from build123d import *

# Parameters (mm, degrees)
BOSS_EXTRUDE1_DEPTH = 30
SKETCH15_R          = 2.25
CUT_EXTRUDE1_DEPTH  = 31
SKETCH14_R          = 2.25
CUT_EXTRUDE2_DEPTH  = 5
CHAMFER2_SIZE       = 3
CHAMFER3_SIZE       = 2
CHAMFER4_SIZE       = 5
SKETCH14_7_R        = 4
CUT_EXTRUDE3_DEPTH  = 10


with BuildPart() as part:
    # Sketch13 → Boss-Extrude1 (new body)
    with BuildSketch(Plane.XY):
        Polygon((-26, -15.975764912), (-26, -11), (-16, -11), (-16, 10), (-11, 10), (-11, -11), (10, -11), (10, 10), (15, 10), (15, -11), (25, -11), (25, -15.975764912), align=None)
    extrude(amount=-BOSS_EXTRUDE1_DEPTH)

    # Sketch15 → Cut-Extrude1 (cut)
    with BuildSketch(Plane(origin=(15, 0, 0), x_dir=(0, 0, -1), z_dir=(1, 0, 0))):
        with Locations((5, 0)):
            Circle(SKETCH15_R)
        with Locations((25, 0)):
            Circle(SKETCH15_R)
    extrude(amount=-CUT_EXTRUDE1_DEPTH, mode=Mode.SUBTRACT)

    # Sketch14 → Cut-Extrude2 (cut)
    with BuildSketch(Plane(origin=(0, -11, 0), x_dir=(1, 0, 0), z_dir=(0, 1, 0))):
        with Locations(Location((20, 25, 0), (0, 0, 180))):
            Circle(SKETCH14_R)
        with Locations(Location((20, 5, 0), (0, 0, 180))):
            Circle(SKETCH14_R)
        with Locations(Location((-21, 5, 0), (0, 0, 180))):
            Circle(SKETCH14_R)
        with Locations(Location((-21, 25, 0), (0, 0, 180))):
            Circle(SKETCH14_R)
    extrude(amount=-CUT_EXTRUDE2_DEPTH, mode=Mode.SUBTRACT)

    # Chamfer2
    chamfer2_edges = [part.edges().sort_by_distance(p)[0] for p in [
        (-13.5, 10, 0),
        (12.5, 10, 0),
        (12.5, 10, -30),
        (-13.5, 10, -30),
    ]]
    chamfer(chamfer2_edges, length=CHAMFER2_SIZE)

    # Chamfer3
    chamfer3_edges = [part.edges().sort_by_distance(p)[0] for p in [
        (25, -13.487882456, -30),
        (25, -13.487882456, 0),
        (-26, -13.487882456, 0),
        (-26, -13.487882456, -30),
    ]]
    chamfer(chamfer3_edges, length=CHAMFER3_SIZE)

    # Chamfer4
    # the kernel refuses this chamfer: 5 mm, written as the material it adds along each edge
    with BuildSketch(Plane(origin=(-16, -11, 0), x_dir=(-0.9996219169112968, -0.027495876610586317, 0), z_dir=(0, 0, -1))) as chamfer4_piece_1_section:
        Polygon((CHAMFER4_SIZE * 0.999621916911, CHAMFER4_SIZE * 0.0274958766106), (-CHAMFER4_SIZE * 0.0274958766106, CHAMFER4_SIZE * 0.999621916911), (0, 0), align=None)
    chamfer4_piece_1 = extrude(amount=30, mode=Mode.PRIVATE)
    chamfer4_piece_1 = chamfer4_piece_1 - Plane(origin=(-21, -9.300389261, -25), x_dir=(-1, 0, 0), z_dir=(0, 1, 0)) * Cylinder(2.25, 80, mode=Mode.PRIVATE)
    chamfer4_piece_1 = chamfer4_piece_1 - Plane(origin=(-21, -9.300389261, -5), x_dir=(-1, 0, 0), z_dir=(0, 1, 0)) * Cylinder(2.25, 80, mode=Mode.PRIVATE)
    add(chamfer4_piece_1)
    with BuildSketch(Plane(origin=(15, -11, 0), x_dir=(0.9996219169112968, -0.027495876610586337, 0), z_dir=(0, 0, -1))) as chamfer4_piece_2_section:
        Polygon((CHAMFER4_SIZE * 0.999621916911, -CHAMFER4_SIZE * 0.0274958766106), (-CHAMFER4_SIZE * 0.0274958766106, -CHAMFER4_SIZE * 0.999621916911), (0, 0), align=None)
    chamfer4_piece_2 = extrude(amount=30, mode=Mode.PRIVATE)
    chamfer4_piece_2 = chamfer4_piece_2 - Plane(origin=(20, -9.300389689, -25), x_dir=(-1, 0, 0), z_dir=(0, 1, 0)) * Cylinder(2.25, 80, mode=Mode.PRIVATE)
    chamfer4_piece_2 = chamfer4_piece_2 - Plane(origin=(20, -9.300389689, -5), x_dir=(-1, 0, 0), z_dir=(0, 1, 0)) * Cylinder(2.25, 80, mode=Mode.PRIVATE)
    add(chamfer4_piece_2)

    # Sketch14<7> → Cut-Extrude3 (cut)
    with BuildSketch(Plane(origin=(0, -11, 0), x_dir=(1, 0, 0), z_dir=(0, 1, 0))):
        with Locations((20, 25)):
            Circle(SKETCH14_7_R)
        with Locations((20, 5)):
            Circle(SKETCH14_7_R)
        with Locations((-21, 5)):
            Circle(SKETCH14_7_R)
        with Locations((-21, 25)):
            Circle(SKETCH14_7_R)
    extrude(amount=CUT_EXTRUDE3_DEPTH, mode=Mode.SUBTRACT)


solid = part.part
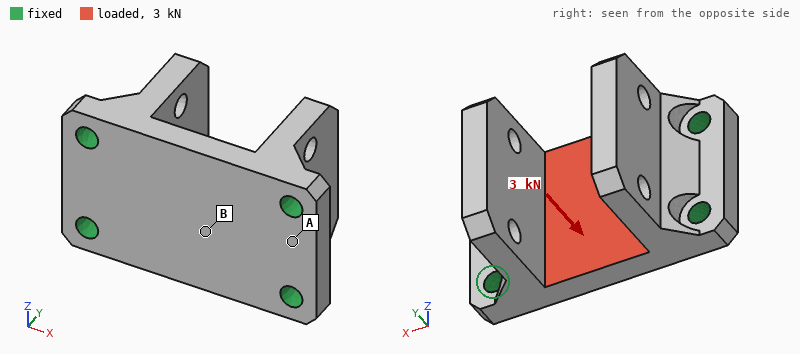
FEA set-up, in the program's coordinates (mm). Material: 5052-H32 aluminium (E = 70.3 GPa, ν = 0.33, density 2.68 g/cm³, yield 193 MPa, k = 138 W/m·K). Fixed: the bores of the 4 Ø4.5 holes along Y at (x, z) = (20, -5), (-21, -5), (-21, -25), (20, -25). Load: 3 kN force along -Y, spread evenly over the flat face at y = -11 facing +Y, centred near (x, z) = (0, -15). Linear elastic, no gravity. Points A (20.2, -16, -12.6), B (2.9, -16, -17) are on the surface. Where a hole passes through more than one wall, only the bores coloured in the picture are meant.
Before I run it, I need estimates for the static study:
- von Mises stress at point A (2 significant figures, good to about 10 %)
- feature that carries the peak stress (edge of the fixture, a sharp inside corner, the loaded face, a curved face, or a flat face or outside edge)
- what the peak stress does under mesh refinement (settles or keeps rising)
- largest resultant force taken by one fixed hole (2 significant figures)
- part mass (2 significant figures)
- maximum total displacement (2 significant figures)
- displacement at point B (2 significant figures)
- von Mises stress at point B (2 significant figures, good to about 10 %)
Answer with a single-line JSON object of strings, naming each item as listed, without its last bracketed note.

{"von Mises stress at point A": "24 MPa", "feature that carries the peak stress": "edge of the fixture", "what the peak stress does under mesh refinement": "keeps rising", "largest resultant force taken by one fixed hole": "750 N", "part mass": "37 g", "maximum total displacement": "55 µm", "displacement at point B": "34 µm", "von Mises stress at point B": "48 MPa"}
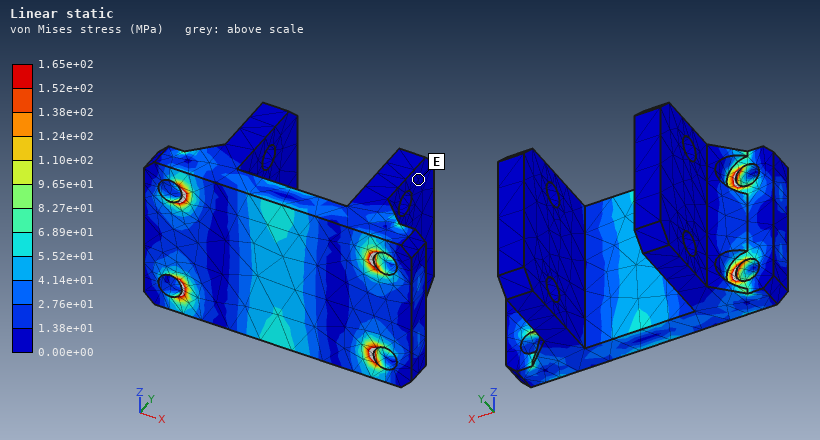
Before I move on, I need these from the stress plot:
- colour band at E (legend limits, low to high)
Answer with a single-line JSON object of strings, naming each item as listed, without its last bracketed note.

{"colour band at E": "0.00e+00 to 1.38e+01 MPa"}
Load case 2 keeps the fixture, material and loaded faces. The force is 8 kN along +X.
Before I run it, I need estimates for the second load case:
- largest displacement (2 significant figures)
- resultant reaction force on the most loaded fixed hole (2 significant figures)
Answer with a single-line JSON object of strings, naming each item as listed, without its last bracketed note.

{"largest displacement": "8.2 µm", "resultant reaction force on the most loaded fixed hole": "2.1 kN"}
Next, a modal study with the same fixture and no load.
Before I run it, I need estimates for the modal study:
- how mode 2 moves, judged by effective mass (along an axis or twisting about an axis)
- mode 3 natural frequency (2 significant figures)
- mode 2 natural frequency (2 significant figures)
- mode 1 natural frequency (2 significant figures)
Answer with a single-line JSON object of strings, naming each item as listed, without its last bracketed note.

{"how mode 2 moves, judged by effective mass": "along X", "mode 3 natural frequency": "14 kHz", "mode 2 natural frequency": "9000 Hz", "mode 1 natural frequency": "7300 Hz"}
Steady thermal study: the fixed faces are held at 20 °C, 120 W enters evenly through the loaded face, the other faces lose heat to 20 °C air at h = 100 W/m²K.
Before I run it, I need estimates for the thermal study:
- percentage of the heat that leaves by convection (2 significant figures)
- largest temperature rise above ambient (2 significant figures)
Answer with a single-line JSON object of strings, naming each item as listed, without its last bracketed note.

{"percentage of the heat that leaves by convection": "7.4 %", "largest temperature rise above ambient": "40 K"}
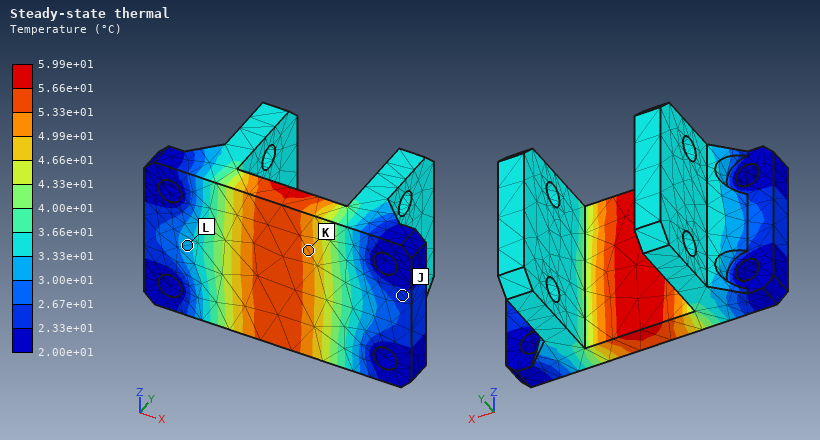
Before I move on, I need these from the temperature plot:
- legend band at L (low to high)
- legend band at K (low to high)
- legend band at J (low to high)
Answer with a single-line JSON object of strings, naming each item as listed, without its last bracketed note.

{"legend band at L": "3.00e+01 to 3.33e+01 °C", "legend band at K": "4.99e+01 to 5.33e+01 °C", "legend band at J": "2.33e+01 to 2.67e+01 °C"}
